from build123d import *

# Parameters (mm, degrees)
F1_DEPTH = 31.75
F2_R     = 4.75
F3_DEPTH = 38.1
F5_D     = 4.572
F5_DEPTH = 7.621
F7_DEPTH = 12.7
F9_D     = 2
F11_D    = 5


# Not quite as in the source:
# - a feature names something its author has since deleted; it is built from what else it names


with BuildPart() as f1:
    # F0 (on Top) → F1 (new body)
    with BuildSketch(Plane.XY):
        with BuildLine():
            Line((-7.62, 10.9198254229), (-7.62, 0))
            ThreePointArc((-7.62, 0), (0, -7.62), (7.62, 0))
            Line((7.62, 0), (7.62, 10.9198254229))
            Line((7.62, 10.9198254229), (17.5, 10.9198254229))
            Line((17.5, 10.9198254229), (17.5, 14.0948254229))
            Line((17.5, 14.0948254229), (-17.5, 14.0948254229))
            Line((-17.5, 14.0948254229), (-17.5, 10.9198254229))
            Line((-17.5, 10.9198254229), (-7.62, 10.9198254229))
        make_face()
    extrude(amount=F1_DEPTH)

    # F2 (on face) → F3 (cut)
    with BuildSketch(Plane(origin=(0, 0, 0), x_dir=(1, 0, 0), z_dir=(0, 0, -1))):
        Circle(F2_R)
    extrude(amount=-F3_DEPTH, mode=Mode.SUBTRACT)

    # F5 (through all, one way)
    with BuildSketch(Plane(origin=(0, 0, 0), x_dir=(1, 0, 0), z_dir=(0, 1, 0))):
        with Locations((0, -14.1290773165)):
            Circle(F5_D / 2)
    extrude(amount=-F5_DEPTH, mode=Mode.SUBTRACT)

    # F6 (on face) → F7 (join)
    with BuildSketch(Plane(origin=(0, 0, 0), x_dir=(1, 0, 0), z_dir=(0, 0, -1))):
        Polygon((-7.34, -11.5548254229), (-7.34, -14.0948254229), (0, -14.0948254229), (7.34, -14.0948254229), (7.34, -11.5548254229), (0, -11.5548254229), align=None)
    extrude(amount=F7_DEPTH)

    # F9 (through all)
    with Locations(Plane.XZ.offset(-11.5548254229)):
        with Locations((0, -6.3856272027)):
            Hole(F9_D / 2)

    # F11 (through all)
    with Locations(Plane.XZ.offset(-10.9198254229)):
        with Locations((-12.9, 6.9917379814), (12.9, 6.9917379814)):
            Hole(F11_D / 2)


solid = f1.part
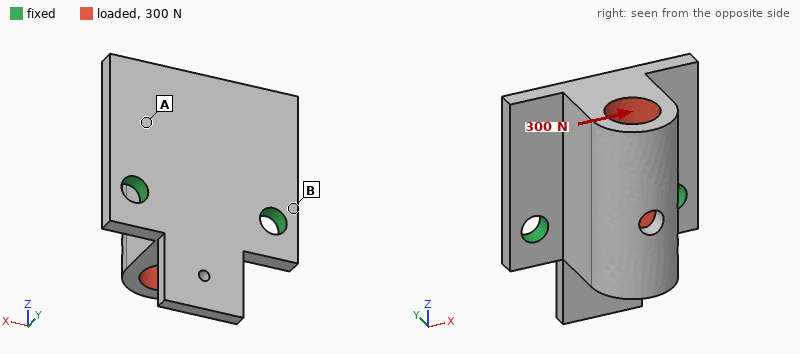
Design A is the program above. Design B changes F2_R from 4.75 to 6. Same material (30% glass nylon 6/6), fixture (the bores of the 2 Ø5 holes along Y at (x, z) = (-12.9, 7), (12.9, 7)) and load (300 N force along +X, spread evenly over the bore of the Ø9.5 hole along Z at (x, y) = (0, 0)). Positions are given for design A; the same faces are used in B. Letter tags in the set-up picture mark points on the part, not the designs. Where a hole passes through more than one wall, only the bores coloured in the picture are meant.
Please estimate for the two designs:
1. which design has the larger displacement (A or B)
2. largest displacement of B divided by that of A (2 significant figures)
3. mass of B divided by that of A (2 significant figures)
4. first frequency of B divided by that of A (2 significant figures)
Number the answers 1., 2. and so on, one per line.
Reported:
1. B
2. 1.5
3. 0.86
4. 1.1
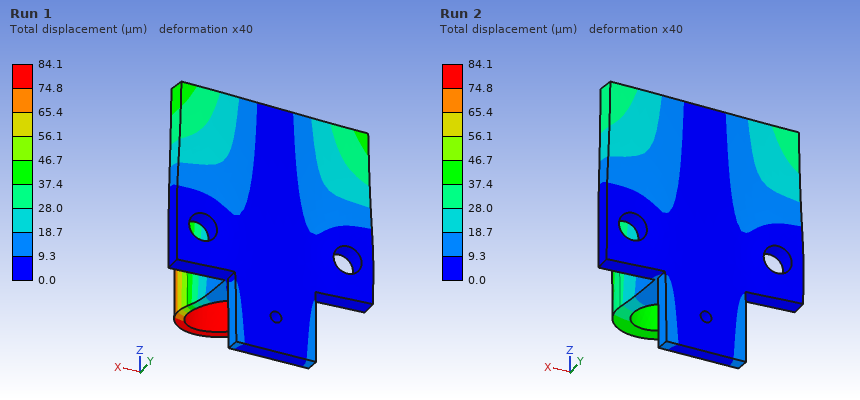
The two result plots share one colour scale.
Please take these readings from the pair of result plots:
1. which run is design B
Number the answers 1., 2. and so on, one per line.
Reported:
1. Run 1
